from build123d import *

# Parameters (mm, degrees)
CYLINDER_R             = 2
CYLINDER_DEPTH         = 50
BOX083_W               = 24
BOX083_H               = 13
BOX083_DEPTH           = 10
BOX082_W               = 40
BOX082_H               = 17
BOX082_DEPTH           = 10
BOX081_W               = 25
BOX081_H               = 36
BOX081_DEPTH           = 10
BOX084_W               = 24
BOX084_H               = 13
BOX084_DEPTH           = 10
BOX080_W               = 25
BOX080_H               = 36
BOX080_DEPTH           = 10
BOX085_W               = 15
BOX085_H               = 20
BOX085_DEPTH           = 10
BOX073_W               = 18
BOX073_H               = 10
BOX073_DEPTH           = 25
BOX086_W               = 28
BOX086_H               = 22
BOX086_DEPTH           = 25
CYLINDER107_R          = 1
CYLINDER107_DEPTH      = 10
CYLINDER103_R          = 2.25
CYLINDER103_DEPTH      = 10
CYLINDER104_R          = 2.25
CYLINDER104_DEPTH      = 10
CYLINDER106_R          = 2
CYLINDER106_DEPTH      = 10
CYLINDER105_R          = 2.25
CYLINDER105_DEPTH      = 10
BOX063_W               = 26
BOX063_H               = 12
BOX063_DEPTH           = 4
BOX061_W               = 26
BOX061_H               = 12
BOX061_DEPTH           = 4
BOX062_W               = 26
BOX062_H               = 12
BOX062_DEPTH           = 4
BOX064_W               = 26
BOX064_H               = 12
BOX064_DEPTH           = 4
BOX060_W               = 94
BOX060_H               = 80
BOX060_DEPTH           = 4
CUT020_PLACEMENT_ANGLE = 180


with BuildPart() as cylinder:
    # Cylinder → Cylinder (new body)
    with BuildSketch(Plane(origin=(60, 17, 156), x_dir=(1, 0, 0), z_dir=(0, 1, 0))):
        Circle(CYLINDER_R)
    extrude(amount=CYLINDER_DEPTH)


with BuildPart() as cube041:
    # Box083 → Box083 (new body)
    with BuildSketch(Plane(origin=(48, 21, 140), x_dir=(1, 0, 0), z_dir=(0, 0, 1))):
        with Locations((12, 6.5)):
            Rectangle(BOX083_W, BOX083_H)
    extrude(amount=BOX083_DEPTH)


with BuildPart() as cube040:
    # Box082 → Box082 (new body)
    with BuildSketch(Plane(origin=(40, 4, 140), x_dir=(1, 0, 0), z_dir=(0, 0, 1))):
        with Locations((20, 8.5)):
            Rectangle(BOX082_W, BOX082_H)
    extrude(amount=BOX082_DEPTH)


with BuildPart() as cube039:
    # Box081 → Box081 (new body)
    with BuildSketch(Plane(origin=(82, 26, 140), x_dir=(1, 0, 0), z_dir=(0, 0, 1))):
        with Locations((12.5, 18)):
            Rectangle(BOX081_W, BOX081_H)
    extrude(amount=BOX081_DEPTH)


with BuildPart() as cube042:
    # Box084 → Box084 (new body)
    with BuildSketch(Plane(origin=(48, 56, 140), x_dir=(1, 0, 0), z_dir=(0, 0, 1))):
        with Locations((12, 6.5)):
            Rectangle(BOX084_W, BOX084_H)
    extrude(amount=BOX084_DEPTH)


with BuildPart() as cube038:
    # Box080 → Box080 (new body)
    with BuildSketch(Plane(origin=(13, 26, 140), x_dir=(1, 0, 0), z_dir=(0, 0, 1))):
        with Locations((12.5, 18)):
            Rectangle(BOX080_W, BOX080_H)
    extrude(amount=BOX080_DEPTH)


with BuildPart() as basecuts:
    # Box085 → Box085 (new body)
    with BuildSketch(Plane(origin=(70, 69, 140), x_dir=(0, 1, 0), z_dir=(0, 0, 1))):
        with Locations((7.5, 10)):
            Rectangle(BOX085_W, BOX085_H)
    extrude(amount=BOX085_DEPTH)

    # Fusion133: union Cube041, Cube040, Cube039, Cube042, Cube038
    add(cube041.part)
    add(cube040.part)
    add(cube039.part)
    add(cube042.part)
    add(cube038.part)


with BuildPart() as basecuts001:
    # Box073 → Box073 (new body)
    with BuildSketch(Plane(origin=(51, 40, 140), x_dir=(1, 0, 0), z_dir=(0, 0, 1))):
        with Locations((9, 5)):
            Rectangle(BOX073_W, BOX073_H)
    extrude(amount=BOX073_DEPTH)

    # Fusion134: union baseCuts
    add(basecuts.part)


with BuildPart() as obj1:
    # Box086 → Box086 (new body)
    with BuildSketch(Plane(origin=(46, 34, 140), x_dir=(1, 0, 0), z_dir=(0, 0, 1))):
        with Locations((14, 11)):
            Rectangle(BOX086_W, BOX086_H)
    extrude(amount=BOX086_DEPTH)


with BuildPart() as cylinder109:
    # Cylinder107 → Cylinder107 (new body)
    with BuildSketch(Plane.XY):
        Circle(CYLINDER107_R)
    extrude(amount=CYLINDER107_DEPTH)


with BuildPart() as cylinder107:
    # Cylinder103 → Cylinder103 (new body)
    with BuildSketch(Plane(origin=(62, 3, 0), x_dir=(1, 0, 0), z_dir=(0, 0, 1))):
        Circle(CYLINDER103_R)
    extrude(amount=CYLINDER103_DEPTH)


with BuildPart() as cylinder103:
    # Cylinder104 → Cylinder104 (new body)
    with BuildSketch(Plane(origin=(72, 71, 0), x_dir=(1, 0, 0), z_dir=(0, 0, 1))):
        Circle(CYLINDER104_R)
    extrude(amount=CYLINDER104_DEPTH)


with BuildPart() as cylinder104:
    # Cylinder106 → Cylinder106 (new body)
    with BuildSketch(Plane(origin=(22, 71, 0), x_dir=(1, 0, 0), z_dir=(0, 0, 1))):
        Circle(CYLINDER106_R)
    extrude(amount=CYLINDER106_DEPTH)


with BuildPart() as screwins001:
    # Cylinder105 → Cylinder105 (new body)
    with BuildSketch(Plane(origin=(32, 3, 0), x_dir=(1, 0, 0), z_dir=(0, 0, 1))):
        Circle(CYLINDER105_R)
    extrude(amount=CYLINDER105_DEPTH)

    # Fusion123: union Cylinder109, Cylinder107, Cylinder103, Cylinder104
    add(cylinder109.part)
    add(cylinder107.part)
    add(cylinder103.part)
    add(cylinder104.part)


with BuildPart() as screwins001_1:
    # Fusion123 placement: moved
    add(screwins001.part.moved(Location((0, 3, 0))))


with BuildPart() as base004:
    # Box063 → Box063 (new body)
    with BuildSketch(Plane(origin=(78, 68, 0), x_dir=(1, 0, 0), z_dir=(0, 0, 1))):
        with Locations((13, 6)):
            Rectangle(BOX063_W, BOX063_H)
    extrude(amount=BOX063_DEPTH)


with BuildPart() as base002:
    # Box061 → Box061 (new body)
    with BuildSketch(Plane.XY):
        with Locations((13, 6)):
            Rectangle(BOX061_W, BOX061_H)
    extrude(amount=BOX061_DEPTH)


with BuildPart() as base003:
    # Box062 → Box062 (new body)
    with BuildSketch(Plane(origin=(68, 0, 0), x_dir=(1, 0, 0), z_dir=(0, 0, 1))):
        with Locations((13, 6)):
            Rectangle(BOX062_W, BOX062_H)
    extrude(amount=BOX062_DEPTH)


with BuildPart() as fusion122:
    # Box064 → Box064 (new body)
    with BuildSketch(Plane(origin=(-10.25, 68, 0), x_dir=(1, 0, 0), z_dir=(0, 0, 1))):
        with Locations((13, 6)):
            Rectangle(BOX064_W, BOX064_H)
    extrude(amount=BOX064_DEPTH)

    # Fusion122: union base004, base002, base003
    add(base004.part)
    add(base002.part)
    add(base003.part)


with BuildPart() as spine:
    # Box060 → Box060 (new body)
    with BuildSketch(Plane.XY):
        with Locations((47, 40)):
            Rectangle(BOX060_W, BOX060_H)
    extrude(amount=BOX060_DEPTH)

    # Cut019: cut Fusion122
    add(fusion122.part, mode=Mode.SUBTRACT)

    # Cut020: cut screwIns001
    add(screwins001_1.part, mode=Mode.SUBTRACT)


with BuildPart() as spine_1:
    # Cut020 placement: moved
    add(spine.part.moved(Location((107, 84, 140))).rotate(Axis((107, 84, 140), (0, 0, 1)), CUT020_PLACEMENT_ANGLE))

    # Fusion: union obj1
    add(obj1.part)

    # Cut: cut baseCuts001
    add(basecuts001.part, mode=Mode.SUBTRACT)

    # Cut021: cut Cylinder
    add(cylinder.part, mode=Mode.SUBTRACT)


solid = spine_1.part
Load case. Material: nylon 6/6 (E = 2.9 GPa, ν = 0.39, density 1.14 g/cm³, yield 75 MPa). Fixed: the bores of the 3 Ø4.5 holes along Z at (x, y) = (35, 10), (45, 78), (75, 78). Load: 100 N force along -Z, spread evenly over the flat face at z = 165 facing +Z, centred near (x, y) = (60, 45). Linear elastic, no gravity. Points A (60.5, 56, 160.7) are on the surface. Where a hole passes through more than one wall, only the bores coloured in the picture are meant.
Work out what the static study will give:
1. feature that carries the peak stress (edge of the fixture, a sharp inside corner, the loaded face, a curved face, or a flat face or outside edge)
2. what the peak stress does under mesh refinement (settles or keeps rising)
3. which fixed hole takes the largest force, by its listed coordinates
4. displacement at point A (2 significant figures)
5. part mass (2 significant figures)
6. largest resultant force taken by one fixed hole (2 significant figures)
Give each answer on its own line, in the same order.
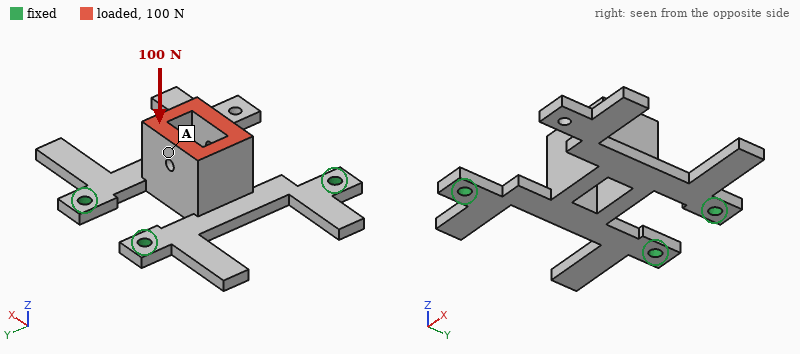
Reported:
edge of the fixture
keeps rising
(75, 78)
0.49 mm
23 g
53 N
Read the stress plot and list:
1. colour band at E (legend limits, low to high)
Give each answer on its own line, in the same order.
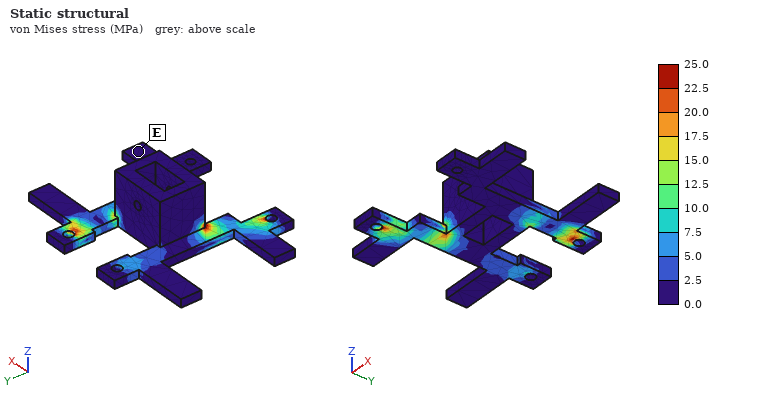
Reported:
0.0 to 2.5 MPa
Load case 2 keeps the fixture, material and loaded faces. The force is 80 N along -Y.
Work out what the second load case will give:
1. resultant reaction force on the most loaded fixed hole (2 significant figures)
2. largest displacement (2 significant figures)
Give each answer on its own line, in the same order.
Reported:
50 N
1.5 mm
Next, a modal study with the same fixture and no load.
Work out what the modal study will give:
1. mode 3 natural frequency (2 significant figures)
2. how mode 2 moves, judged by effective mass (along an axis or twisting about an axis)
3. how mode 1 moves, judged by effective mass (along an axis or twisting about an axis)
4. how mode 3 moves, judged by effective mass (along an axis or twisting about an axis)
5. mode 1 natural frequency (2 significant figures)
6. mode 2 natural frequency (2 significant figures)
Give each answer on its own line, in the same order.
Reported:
820 Hz
along Z
along Z
along X
310 Hz
710 Hz
